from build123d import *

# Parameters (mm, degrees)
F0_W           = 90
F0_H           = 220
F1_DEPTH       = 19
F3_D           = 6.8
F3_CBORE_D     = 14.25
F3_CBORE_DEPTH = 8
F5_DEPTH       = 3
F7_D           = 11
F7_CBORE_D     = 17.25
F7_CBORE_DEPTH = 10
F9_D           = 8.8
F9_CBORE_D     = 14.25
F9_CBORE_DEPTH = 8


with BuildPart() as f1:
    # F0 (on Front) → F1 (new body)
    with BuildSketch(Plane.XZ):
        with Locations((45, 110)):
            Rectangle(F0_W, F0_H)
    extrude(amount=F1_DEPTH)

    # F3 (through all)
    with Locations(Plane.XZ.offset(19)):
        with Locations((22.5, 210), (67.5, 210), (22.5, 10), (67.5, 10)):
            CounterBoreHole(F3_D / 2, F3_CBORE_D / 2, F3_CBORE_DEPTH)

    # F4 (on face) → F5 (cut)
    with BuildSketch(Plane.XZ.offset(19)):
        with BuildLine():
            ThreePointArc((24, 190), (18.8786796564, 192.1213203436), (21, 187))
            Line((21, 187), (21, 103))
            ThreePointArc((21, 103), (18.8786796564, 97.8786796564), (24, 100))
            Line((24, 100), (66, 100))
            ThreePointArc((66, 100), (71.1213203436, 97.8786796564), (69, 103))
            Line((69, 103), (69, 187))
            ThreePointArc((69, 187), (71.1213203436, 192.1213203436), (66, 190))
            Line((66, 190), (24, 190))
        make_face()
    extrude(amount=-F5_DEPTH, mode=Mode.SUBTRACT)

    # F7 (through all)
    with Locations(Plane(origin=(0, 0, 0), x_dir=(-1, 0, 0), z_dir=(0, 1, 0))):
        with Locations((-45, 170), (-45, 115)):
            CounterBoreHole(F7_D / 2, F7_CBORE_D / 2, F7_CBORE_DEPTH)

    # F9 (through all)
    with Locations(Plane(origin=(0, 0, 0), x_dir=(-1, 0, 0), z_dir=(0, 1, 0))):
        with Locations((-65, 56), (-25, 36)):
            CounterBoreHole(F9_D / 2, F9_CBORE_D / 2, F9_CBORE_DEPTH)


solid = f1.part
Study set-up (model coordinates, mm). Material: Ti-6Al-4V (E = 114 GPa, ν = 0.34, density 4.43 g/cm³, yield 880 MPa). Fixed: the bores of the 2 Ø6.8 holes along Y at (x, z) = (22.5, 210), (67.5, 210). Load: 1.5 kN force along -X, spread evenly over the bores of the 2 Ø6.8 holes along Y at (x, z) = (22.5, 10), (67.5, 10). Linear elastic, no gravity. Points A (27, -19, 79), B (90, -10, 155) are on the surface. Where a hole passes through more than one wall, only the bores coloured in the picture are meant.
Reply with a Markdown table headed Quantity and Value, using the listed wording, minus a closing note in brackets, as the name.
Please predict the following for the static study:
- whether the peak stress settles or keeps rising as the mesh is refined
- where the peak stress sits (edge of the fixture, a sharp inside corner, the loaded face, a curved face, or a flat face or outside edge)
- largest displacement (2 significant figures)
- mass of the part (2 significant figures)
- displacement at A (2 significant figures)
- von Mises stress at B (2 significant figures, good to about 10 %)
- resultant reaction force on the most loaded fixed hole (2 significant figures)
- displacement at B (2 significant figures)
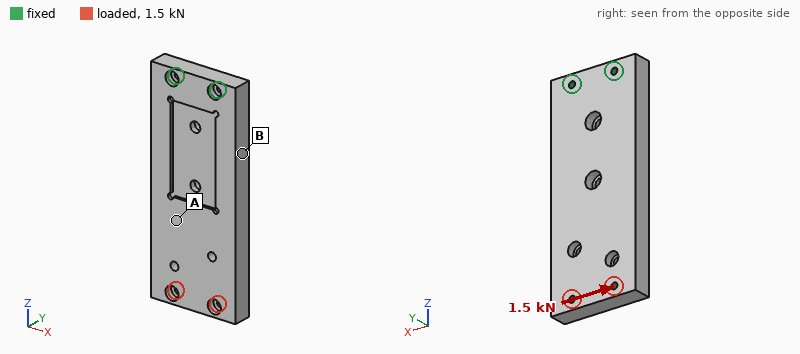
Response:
| Quantity | Value |
|---|---|
| whether the peak stress settles or keeps rising as the mesh is refined | keeps rising |
| where the peak stress sits | edge of the fixture |
| largest displacement | 72 µm |
| mass of the part | 1.5 kg |
| displacement at A | 35 µm |
| von Mises stress at B | 8.3 MPa |
| resultant reaction force on the most loaded fixed hole | 6.2 kN |
| displacement at B | 18 µm |
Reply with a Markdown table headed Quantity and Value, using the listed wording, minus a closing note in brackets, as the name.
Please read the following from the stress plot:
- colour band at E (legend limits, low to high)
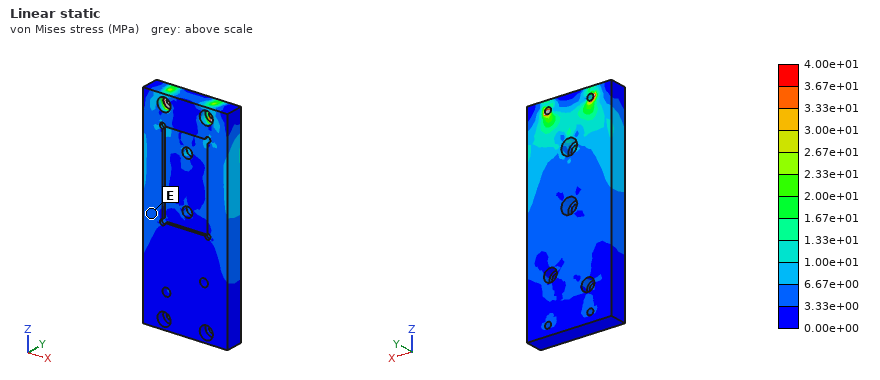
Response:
| Quantity | Value |
|---|---|
| colour band at E | 3.33e+00 to 6.67e+00 MPa |
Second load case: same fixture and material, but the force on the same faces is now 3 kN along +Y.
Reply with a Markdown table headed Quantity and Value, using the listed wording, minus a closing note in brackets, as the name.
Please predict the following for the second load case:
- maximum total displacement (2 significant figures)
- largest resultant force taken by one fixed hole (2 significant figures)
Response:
| Quantity | Value |
|---|---|
| maximum total displacement | 2.6 mm |
| largest resultant force taken by one fixed hole | 2.7 kN |
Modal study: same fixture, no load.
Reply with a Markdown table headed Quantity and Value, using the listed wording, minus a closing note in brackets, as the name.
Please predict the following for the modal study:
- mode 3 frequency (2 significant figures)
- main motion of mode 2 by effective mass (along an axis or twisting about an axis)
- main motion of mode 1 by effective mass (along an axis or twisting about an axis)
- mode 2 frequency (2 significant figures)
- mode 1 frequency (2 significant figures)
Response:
| Quantity | Value |
|---|---|
| mode 3 frequency | 1300 Hz |
| main motion of mode 2 by effective mass | along X |
| main motion of mode 1 by effective mass | along Y |
| mode 2 frequency | 1100 Hz |
| mode 1 frequency | 260 Hz |
